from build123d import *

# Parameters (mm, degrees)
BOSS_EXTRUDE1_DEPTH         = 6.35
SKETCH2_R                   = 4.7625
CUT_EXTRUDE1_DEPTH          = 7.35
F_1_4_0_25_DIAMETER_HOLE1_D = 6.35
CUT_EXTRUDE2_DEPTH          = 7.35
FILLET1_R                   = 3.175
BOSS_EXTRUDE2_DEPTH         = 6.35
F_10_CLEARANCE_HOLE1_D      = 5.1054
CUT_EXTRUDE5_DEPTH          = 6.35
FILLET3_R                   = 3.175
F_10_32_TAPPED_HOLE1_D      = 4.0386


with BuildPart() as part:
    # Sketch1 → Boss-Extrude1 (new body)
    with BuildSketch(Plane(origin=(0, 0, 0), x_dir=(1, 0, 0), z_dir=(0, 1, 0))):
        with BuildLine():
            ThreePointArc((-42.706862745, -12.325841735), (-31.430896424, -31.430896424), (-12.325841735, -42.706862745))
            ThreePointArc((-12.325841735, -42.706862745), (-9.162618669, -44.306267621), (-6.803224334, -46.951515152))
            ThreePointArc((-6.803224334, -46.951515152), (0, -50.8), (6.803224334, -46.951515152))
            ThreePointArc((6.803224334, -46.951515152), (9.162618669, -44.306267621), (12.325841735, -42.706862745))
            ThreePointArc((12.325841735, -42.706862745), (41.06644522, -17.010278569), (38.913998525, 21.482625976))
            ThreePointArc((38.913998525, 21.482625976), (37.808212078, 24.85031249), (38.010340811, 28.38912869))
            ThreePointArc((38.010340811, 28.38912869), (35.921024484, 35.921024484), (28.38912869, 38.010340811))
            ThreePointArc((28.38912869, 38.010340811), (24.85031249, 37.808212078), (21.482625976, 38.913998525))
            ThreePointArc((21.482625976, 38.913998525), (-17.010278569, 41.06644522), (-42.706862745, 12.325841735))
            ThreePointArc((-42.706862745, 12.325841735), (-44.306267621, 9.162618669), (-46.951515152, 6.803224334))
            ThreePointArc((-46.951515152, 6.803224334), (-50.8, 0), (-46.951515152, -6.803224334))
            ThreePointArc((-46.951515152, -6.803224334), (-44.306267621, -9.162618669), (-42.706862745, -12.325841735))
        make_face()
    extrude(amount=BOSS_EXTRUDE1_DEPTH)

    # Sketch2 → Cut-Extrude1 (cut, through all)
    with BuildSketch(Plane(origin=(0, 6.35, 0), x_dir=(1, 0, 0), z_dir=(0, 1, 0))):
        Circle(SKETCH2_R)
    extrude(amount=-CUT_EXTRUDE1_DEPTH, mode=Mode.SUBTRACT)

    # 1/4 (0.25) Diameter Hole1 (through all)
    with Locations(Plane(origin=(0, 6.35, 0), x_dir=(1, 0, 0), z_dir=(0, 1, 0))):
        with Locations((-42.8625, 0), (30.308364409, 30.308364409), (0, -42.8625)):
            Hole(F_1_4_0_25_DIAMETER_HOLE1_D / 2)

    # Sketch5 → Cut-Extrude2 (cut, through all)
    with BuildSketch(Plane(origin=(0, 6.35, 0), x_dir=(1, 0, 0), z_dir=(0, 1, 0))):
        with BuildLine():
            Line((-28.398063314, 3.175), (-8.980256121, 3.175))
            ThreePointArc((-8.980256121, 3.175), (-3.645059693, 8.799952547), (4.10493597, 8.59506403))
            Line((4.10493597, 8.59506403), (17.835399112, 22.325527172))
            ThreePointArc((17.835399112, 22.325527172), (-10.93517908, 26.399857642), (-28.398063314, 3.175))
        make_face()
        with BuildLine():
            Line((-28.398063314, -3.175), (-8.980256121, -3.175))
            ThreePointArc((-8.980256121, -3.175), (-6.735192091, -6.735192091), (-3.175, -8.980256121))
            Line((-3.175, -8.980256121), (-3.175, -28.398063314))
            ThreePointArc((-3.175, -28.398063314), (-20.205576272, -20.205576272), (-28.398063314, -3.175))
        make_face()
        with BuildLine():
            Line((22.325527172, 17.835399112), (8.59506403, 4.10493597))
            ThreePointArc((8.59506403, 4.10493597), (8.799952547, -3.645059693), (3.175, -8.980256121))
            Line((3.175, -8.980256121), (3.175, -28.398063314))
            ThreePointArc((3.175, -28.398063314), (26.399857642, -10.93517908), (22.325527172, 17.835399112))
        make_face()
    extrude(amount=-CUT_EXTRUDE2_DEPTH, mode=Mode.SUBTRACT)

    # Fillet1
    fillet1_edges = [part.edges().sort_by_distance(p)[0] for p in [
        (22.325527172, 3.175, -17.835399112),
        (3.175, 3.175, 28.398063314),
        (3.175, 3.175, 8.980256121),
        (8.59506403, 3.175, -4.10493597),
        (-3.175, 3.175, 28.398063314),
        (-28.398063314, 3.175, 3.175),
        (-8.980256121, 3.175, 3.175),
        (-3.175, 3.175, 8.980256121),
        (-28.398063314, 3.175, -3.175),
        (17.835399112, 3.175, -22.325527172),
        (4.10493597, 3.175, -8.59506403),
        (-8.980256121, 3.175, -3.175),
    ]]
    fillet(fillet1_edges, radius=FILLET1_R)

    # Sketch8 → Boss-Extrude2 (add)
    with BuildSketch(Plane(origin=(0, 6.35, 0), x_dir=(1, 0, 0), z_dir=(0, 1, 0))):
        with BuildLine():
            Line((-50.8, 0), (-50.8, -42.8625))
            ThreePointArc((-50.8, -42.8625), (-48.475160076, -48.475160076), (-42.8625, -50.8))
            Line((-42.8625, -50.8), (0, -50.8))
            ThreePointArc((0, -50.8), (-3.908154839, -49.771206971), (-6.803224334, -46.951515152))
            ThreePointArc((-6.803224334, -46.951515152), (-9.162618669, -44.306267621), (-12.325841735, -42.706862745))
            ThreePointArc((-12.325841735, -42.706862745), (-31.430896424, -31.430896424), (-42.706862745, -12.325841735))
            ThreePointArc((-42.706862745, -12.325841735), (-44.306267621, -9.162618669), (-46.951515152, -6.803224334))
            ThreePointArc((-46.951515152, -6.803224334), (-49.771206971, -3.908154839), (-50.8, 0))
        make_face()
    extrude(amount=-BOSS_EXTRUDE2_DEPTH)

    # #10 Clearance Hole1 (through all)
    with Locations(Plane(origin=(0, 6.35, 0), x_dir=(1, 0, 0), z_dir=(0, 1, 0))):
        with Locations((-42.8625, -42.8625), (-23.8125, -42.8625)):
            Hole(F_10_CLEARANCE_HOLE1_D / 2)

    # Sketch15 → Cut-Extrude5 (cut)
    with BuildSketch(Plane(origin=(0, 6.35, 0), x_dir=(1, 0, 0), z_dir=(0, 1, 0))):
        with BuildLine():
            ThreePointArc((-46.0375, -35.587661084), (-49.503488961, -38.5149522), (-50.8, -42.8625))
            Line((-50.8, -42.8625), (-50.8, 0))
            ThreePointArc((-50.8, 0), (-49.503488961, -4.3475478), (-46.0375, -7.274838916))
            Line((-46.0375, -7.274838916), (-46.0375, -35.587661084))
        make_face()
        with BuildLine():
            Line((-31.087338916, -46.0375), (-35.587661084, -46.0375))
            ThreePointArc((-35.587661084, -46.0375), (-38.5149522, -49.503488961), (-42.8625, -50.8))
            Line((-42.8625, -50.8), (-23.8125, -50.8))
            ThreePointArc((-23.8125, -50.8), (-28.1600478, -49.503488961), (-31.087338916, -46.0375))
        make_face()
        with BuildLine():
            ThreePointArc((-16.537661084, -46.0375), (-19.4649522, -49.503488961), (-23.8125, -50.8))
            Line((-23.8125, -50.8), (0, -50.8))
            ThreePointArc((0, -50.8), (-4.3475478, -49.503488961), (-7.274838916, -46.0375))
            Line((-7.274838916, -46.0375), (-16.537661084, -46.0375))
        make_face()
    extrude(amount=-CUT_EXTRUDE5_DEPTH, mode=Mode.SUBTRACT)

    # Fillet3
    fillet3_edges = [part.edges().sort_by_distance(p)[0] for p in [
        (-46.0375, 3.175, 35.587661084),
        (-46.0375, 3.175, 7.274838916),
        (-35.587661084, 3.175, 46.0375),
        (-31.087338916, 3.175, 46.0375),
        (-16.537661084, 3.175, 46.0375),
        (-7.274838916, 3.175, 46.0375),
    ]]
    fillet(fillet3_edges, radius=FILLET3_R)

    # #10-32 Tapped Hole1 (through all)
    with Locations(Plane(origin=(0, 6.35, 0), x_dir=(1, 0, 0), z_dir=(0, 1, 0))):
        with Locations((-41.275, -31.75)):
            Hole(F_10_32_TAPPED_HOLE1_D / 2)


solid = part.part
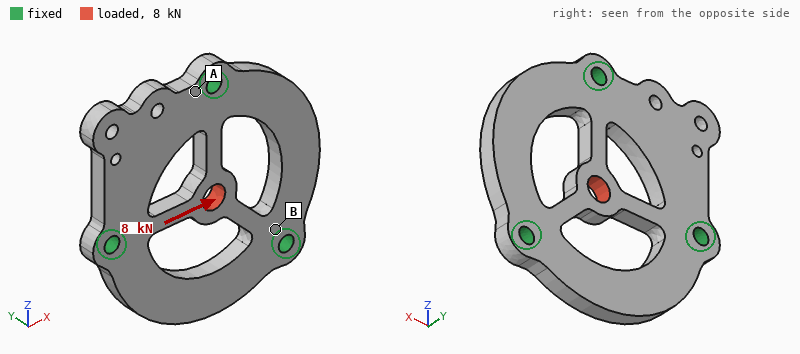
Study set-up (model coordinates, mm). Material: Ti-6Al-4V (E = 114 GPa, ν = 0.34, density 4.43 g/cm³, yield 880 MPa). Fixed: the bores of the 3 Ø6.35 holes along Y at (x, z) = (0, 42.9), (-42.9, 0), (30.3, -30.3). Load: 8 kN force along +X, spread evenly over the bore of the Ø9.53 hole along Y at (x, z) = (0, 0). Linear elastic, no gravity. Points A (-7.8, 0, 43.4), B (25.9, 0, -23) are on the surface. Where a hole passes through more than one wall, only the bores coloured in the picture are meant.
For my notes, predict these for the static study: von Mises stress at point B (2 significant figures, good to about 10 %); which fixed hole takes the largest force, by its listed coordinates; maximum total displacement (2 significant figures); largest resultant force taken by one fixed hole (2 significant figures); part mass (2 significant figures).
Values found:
46 MPa
(-42.9, 0)
66 µm
5.1 kN
140 g
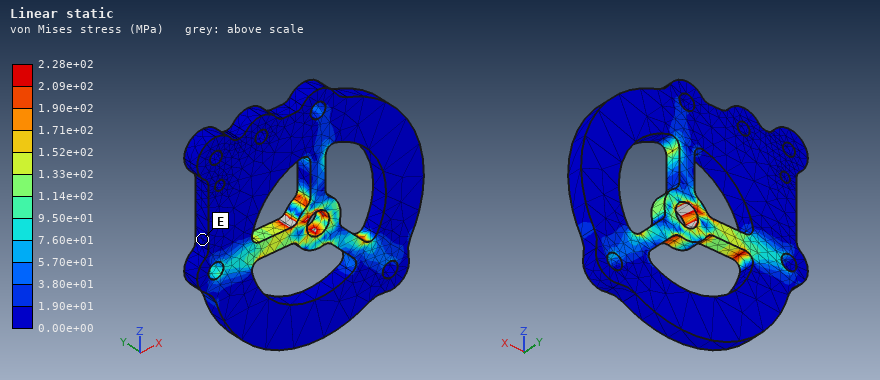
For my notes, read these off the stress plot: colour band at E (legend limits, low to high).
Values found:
0.00e+00 to 1.90e+01 MPa
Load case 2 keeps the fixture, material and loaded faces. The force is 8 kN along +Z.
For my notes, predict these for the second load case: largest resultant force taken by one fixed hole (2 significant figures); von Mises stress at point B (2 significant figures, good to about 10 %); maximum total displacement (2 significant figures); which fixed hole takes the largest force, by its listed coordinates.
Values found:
5.1 kN
26 MPa
66 µm
(0, 42.9)
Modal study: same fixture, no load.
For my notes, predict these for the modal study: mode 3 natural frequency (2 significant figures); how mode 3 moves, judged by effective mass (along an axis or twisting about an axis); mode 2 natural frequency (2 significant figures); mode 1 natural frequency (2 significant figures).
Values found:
4000 Hz
along Y
3800 Hz
3600 Hz
